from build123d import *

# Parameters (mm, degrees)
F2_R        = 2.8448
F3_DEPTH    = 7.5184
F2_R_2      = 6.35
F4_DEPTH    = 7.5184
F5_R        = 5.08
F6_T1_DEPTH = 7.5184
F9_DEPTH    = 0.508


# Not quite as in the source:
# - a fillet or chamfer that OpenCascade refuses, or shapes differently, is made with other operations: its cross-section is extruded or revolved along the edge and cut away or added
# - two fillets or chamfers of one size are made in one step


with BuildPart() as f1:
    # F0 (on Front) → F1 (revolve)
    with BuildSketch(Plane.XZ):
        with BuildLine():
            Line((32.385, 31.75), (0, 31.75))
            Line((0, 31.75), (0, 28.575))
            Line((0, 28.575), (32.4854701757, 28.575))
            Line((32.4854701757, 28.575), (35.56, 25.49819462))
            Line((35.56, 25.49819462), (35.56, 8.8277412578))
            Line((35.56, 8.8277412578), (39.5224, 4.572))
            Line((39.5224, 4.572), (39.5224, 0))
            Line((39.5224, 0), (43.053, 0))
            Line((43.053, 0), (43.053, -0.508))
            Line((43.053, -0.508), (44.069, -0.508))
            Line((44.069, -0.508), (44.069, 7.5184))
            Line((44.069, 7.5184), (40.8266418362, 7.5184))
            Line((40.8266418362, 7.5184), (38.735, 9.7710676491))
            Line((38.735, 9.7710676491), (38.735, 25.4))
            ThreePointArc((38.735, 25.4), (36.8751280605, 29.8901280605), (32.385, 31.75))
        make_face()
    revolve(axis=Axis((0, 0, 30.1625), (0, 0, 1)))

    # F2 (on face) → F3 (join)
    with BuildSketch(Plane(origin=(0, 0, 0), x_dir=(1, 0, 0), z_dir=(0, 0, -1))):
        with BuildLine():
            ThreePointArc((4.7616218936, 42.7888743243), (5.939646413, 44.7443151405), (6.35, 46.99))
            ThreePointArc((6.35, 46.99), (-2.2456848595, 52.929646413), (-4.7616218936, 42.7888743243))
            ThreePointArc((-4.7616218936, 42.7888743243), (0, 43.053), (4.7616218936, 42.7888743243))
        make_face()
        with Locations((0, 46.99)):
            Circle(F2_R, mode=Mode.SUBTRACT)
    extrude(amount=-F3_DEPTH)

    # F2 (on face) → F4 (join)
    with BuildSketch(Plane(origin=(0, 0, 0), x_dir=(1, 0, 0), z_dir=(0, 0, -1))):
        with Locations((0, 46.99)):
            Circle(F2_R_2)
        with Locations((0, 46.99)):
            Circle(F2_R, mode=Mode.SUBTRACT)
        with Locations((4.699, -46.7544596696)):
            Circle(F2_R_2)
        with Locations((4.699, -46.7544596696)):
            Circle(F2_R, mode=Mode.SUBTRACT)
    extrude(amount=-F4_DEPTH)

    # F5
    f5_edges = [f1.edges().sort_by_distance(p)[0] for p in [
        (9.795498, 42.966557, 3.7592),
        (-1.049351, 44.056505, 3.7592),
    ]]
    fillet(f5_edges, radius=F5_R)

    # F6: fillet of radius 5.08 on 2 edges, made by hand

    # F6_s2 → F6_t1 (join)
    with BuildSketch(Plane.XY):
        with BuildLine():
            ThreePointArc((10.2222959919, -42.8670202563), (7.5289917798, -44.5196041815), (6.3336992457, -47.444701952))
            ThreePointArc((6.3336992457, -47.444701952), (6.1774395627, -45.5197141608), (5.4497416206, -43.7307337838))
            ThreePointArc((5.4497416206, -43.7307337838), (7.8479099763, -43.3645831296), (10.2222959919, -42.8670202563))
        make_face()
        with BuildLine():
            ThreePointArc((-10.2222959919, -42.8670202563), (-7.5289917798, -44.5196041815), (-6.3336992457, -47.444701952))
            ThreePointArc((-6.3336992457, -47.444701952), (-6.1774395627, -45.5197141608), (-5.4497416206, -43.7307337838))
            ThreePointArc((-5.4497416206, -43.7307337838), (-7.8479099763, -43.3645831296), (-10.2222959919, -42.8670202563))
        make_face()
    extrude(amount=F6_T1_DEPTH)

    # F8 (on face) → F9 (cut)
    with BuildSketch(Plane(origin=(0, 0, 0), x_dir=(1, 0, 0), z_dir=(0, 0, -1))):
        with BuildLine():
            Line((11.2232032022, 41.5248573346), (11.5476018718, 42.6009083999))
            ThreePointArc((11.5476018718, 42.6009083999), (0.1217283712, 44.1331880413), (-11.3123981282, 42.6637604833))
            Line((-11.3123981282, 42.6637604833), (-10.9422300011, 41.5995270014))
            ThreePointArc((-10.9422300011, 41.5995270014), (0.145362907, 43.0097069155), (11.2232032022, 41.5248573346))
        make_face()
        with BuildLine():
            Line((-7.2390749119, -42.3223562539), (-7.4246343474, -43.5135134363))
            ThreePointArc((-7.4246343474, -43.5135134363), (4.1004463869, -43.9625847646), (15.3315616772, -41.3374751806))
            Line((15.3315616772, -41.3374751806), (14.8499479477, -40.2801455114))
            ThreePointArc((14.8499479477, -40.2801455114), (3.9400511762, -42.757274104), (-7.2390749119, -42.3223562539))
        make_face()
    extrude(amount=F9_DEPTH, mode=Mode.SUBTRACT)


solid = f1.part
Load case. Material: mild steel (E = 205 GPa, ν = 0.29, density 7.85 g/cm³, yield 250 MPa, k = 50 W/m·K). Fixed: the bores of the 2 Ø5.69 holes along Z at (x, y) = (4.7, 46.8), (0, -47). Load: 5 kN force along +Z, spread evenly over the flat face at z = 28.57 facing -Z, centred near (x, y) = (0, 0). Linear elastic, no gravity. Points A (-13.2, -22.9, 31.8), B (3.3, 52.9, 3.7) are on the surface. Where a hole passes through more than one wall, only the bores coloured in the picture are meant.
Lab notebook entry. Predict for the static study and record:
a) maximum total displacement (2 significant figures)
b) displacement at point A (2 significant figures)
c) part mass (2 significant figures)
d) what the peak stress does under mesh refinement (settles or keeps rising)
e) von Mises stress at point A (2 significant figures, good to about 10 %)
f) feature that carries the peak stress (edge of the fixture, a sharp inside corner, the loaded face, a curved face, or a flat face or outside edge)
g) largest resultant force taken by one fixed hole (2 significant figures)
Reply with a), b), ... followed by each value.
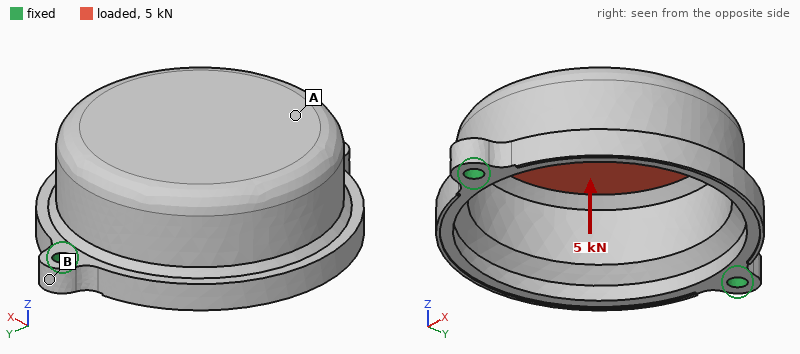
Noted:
a) 92 µm
b) 37 µm
c) 320 g
d) keeps rising
e) 43 MPa
f) edge of the fixture
g) 2.9 kN
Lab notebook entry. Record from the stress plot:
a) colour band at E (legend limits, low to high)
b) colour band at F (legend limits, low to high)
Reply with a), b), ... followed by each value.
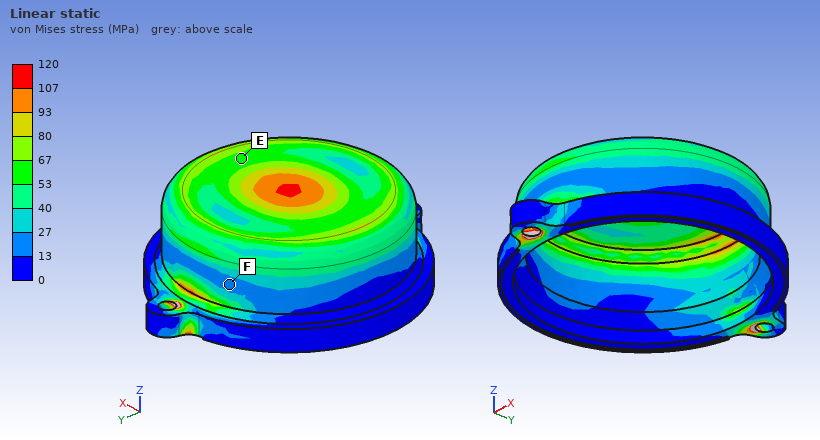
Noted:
a) 53 to 67 MPa
b) 13 to 27 MPa
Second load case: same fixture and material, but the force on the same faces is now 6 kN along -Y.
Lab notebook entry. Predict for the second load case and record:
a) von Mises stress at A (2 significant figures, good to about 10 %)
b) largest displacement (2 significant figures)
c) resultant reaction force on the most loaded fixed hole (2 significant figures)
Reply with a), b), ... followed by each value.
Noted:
a) 19 MPa
b) 58 µm
c) 3.5 kN
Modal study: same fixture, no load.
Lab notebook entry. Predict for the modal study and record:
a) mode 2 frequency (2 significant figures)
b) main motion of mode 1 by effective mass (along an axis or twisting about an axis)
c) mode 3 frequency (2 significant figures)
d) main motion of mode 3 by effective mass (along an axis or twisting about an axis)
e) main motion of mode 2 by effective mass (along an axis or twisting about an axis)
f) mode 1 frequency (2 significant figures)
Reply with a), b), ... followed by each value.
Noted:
a) 3400 Hz
b) along X
c) 4000 Hz
d) along Y
e) along Y
f) 1600 Hz
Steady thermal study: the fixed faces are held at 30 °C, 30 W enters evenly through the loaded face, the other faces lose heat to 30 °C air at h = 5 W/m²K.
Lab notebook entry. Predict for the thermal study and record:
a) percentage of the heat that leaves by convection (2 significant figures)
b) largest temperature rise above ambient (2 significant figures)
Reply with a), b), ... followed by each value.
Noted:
a) 17 %
b) 71 K
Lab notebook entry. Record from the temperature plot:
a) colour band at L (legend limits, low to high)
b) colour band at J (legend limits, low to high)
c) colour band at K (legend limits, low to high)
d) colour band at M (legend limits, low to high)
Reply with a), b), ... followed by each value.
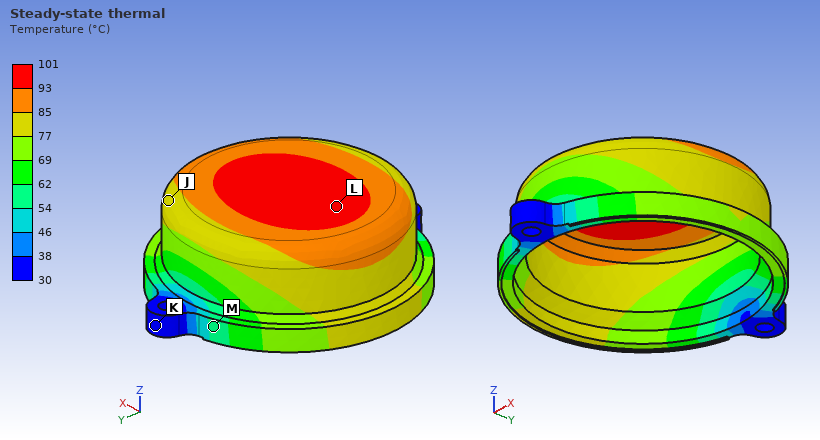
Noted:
a) 93 to 101 °C
b) 77 to 85 °C
c) 30 to 38 °C
d) 54 to 62 °C
